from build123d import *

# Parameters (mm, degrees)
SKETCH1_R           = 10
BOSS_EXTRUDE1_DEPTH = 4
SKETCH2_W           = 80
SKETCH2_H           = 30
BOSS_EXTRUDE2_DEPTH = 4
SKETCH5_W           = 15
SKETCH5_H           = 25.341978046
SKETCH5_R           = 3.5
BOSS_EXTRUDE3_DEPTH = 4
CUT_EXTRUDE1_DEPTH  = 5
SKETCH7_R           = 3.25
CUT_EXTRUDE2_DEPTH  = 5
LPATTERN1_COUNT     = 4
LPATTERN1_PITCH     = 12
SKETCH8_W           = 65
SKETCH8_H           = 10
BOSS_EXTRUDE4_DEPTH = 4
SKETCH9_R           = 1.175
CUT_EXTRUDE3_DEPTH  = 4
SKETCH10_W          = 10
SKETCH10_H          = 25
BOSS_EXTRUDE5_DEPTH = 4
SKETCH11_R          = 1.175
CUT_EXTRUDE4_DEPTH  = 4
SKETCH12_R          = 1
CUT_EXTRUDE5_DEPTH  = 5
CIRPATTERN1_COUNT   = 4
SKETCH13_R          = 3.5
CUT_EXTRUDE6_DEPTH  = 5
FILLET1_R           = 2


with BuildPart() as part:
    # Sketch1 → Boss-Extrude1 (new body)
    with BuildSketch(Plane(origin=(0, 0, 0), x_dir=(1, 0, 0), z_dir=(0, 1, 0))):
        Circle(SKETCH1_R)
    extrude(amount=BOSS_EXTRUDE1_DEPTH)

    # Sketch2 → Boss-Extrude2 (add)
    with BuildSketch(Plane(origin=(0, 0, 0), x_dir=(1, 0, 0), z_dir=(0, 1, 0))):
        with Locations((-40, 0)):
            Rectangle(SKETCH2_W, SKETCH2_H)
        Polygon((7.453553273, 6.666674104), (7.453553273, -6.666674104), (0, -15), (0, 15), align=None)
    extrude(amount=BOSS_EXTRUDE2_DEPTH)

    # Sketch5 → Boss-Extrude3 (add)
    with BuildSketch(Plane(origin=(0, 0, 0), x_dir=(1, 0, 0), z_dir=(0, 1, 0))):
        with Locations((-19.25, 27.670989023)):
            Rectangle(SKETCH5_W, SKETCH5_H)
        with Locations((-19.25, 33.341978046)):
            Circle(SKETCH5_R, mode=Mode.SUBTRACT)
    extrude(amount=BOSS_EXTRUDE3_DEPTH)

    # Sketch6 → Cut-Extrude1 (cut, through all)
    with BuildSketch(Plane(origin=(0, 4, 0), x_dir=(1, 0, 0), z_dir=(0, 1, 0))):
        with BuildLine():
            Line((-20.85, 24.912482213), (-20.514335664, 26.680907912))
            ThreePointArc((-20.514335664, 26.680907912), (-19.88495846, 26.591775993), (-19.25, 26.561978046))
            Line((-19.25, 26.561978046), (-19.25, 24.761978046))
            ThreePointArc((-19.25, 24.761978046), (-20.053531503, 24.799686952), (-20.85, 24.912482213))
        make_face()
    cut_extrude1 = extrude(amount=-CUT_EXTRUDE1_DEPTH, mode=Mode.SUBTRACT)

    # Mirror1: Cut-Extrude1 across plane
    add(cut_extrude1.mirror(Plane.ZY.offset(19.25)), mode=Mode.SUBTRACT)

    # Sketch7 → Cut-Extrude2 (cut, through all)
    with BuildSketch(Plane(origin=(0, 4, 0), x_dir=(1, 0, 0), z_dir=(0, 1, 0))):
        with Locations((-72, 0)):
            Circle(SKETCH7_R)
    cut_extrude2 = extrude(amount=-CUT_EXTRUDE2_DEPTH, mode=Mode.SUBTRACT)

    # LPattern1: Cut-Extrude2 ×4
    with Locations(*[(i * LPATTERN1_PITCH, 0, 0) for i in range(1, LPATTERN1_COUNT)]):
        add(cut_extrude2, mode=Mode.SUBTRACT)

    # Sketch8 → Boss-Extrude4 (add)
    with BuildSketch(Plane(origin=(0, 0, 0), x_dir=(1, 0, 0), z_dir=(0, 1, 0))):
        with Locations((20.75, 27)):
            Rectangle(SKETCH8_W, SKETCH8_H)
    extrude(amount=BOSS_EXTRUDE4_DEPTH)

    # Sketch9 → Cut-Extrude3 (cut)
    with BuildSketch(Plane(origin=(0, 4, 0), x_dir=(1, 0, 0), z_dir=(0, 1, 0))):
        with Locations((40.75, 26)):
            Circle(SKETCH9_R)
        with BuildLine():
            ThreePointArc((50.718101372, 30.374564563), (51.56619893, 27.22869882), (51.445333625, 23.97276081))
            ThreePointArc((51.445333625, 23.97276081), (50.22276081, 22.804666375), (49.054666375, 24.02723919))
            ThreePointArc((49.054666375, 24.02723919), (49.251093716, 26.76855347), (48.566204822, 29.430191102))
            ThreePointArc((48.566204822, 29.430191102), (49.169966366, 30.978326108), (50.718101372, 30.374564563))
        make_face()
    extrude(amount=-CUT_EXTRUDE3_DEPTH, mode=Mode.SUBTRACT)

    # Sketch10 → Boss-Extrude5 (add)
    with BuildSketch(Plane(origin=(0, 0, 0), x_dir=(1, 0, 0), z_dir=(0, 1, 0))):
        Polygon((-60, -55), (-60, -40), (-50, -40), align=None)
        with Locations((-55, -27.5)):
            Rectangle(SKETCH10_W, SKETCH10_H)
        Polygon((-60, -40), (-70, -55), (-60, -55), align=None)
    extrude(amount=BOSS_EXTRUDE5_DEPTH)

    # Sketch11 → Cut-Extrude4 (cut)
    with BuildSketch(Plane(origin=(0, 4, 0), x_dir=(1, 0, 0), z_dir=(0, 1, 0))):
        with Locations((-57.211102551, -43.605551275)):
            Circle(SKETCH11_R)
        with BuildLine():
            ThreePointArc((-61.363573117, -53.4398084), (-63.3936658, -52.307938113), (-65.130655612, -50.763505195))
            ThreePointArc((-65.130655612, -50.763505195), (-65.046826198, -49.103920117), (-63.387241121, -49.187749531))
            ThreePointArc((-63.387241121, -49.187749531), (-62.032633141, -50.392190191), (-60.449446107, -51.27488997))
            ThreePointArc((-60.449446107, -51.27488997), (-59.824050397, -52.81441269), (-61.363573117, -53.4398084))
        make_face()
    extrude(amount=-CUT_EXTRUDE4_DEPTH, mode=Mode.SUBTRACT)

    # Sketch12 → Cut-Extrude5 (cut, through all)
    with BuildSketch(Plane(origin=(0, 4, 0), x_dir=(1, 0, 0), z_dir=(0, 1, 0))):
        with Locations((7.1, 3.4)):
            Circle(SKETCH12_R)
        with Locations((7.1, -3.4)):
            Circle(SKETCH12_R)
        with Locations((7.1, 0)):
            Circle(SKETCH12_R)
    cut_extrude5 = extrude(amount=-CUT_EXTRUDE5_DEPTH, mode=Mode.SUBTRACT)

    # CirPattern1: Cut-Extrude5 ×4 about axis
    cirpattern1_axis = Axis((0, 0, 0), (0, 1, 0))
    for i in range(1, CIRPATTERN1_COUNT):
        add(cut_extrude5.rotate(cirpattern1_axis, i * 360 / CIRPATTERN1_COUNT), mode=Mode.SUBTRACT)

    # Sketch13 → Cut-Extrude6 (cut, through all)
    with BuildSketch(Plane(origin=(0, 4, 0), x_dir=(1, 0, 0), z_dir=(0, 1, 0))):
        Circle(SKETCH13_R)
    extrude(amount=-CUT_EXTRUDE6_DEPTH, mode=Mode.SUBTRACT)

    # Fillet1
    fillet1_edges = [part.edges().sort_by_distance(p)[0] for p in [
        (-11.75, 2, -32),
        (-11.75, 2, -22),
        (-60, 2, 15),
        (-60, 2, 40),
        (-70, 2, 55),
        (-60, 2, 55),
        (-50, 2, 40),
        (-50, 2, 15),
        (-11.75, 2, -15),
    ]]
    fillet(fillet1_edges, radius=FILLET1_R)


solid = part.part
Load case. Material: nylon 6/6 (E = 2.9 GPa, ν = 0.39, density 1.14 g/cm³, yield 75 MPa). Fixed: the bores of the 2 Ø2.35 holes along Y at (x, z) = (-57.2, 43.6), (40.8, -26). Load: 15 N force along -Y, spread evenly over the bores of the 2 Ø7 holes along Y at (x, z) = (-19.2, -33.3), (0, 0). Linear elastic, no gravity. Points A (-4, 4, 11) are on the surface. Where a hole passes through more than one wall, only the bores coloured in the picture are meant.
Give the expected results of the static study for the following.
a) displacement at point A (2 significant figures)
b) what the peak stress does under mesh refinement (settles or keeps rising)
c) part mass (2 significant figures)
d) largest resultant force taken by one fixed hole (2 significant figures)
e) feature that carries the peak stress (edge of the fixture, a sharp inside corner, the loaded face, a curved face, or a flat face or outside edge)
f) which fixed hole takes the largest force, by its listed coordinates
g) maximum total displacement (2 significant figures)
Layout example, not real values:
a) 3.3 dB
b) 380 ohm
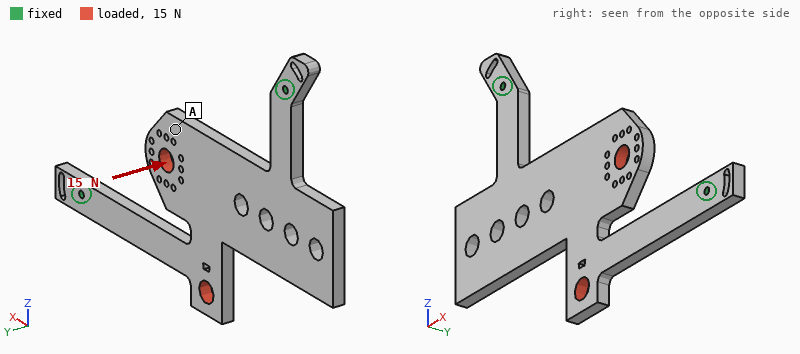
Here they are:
a) 0.88 mm
b) keeps rising
c) 17 g
d) 9.9 N
e) edge of the fixture
f) (40.8, -26)
g) 1.6 mm
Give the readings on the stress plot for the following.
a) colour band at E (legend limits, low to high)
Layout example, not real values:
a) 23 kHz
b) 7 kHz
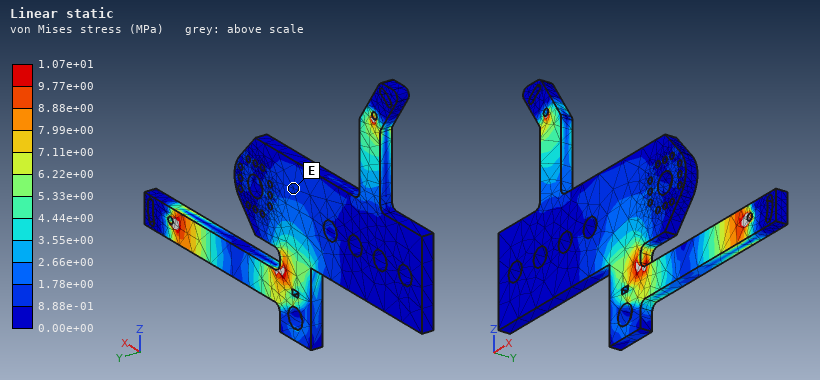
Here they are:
a) 8.88e-01 to 1.78e+00 MPa
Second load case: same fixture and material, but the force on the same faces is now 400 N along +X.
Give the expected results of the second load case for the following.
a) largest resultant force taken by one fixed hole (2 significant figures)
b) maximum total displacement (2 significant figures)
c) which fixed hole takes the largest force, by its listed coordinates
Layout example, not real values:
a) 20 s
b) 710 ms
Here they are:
a) 340 N
b) 0.42 mm
c) (40.8, -26)
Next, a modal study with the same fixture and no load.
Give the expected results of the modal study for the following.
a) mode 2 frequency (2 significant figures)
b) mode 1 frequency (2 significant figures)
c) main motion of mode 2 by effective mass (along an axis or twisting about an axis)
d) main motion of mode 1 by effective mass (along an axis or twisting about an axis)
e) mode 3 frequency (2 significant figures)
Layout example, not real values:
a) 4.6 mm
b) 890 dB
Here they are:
a) 250 Hz
b) 170 Hz
c) along Y
d) along Y
e) 530 Hz
